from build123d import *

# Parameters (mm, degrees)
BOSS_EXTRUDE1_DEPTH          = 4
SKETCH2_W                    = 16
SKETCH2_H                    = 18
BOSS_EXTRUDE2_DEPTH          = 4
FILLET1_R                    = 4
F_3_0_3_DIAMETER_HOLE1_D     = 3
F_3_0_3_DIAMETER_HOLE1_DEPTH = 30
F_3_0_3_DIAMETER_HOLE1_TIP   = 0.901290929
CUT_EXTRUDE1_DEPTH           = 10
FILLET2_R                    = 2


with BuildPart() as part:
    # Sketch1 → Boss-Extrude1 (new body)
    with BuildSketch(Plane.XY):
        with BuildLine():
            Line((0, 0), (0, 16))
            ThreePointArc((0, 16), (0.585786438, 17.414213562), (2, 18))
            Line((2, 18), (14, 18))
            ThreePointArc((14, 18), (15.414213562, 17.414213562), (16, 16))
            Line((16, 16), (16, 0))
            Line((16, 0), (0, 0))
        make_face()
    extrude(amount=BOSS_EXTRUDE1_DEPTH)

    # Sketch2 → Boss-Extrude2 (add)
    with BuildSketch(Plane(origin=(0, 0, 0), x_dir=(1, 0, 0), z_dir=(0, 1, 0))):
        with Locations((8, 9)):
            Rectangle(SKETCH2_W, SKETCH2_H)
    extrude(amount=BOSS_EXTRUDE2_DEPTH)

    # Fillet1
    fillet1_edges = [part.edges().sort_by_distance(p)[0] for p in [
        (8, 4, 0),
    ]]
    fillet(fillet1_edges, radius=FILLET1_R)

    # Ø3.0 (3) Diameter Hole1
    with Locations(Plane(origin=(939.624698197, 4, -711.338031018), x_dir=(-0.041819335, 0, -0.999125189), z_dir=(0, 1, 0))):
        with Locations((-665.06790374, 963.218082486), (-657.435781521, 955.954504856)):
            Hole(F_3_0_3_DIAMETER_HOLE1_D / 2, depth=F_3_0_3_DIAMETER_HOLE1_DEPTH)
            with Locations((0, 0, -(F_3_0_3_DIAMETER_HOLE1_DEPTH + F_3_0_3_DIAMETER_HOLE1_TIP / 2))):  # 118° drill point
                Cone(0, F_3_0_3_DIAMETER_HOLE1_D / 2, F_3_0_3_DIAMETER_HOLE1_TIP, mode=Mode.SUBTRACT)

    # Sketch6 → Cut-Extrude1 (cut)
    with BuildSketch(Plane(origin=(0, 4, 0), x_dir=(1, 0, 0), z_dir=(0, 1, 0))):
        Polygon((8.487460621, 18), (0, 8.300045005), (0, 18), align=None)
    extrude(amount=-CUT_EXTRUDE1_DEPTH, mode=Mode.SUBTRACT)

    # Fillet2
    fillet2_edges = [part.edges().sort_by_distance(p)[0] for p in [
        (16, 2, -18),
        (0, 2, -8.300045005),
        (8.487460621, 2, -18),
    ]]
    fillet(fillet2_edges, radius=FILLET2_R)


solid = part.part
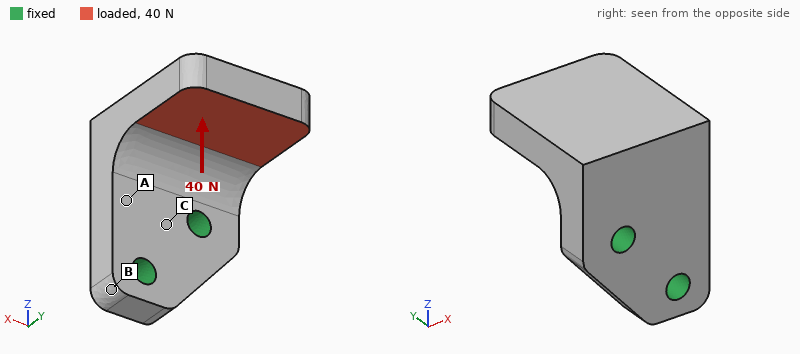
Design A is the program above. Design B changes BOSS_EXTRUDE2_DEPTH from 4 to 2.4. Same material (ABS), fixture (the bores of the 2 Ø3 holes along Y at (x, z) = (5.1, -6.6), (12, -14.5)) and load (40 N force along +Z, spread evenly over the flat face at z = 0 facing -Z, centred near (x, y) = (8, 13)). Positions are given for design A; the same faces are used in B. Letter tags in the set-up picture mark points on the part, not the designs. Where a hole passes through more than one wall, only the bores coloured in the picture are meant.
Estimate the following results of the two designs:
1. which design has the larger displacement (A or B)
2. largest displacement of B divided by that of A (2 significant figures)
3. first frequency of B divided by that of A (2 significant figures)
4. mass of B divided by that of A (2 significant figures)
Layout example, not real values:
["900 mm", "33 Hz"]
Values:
["B", "3.3", "0.51", "0.83"]
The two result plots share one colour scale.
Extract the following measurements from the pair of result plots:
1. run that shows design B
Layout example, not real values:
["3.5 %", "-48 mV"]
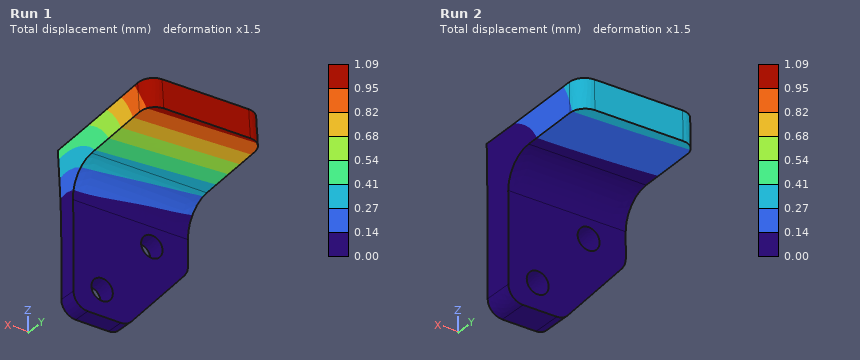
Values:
["Run 1"]
